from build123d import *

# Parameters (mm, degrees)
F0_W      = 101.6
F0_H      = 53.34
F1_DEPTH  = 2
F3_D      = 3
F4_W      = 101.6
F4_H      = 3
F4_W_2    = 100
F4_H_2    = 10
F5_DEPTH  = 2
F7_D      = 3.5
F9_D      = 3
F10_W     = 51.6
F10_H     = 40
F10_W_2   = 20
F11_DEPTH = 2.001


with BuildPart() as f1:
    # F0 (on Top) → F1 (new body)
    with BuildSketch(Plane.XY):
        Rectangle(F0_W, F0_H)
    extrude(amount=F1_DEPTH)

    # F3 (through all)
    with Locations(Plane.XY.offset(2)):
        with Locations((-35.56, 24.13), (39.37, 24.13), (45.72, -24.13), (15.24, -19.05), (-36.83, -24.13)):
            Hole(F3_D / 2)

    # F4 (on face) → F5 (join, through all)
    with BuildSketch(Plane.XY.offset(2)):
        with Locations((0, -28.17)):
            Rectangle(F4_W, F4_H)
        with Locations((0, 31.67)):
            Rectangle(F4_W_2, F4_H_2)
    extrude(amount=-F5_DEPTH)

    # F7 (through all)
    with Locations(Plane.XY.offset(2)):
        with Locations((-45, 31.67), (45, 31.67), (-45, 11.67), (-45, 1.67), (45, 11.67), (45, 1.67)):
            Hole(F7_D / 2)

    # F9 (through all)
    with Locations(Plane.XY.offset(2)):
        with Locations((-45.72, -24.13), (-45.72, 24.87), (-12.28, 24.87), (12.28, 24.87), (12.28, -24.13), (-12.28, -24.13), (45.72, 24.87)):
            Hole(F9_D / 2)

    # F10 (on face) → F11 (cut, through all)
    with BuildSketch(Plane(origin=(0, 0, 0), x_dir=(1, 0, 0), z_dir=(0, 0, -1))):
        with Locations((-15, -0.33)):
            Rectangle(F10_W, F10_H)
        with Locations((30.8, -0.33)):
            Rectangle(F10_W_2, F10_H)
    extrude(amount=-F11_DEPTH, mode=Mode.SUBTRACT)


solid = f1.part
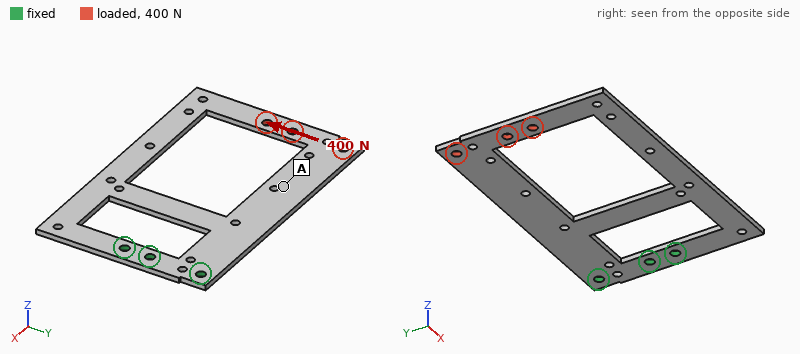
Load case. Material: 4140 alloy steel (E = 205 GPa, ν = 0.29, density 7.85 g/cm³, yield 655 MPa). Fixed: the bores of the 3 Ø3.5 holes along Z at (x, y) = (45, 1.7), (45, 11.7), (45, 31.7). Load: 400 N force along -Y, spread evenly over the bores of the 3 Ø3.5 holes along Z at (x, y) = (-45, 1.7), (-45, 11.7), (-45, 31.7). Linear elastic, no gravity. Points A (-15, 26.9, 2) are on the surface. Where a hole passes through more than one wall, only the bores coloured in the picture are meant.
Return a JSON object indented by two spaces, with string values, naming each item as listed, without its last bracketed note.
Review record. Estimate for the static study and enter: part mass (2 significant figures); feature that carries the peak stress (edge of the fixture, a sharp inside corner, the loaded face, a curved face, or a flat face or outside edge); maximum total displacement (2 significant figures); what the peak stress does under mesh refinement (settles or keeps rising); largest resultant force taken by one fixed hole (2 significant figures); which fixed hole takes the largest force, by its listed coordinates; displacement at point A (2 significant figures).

{
  "part mass": "58 g",
  "feature that carries the peak stress": "a sharp inside corner",
  "maximum total displacement": "0.28 mm",
  "what the peak stress does under mesh refinement": "keeps rising",
  "largest resultant force taken by one fixed hole": "1.2 kN",
  "which fixed hole takes the largest force, by its listed coordinates": "(45, 31.7)",
  "displacement at point A": "0.15 mm"
}
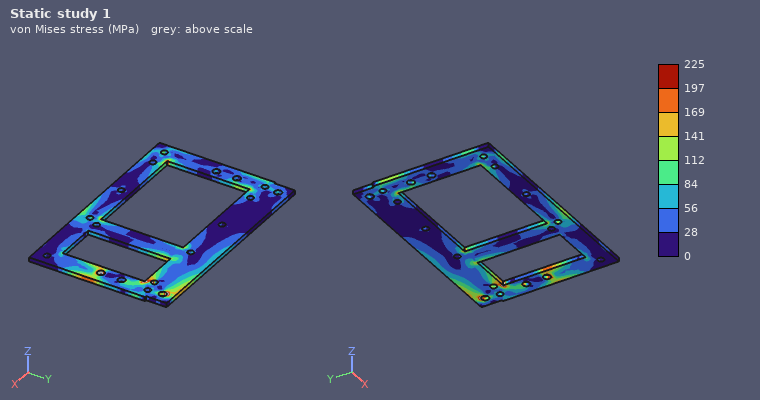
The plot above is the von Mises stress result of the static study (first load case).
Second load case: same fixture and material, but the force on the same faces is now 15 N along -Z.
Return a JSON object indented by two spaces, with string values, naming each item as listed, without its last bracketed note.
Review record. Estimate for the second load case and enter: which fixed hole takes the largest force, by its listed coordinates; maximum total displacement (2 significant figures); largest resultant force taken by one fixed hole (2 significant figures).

{
  "which fixed hole takes the largest force, by its listed coordinates": "(45, 31.7)",
  "maximum total displacement": "1.3 mm",
  "largest resultant force taken by one fixed hole": "16 N"
}
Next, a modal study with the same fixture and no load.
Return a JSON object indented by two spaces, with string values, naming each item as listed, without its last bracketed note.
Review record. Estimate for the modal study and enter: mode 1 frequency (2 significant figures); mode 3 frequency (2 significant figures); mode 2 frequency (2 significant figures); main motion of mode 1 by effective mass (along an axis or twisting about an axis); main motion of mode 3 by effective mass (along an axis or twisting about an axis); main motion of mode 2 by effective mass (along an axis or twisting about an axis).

{
  "mode 1 frequency": "140 Hz",
  "mode 3 frequency": "770 Hz",
  "mode 2 frequency": "390 Hz",
  "main motion of mode 1 by effective mass": "along Z",
  "main motion of mode 3 by effective mass": "along Z",
  "main motion of mode 2 by effective mass": "twisting about X"
}
